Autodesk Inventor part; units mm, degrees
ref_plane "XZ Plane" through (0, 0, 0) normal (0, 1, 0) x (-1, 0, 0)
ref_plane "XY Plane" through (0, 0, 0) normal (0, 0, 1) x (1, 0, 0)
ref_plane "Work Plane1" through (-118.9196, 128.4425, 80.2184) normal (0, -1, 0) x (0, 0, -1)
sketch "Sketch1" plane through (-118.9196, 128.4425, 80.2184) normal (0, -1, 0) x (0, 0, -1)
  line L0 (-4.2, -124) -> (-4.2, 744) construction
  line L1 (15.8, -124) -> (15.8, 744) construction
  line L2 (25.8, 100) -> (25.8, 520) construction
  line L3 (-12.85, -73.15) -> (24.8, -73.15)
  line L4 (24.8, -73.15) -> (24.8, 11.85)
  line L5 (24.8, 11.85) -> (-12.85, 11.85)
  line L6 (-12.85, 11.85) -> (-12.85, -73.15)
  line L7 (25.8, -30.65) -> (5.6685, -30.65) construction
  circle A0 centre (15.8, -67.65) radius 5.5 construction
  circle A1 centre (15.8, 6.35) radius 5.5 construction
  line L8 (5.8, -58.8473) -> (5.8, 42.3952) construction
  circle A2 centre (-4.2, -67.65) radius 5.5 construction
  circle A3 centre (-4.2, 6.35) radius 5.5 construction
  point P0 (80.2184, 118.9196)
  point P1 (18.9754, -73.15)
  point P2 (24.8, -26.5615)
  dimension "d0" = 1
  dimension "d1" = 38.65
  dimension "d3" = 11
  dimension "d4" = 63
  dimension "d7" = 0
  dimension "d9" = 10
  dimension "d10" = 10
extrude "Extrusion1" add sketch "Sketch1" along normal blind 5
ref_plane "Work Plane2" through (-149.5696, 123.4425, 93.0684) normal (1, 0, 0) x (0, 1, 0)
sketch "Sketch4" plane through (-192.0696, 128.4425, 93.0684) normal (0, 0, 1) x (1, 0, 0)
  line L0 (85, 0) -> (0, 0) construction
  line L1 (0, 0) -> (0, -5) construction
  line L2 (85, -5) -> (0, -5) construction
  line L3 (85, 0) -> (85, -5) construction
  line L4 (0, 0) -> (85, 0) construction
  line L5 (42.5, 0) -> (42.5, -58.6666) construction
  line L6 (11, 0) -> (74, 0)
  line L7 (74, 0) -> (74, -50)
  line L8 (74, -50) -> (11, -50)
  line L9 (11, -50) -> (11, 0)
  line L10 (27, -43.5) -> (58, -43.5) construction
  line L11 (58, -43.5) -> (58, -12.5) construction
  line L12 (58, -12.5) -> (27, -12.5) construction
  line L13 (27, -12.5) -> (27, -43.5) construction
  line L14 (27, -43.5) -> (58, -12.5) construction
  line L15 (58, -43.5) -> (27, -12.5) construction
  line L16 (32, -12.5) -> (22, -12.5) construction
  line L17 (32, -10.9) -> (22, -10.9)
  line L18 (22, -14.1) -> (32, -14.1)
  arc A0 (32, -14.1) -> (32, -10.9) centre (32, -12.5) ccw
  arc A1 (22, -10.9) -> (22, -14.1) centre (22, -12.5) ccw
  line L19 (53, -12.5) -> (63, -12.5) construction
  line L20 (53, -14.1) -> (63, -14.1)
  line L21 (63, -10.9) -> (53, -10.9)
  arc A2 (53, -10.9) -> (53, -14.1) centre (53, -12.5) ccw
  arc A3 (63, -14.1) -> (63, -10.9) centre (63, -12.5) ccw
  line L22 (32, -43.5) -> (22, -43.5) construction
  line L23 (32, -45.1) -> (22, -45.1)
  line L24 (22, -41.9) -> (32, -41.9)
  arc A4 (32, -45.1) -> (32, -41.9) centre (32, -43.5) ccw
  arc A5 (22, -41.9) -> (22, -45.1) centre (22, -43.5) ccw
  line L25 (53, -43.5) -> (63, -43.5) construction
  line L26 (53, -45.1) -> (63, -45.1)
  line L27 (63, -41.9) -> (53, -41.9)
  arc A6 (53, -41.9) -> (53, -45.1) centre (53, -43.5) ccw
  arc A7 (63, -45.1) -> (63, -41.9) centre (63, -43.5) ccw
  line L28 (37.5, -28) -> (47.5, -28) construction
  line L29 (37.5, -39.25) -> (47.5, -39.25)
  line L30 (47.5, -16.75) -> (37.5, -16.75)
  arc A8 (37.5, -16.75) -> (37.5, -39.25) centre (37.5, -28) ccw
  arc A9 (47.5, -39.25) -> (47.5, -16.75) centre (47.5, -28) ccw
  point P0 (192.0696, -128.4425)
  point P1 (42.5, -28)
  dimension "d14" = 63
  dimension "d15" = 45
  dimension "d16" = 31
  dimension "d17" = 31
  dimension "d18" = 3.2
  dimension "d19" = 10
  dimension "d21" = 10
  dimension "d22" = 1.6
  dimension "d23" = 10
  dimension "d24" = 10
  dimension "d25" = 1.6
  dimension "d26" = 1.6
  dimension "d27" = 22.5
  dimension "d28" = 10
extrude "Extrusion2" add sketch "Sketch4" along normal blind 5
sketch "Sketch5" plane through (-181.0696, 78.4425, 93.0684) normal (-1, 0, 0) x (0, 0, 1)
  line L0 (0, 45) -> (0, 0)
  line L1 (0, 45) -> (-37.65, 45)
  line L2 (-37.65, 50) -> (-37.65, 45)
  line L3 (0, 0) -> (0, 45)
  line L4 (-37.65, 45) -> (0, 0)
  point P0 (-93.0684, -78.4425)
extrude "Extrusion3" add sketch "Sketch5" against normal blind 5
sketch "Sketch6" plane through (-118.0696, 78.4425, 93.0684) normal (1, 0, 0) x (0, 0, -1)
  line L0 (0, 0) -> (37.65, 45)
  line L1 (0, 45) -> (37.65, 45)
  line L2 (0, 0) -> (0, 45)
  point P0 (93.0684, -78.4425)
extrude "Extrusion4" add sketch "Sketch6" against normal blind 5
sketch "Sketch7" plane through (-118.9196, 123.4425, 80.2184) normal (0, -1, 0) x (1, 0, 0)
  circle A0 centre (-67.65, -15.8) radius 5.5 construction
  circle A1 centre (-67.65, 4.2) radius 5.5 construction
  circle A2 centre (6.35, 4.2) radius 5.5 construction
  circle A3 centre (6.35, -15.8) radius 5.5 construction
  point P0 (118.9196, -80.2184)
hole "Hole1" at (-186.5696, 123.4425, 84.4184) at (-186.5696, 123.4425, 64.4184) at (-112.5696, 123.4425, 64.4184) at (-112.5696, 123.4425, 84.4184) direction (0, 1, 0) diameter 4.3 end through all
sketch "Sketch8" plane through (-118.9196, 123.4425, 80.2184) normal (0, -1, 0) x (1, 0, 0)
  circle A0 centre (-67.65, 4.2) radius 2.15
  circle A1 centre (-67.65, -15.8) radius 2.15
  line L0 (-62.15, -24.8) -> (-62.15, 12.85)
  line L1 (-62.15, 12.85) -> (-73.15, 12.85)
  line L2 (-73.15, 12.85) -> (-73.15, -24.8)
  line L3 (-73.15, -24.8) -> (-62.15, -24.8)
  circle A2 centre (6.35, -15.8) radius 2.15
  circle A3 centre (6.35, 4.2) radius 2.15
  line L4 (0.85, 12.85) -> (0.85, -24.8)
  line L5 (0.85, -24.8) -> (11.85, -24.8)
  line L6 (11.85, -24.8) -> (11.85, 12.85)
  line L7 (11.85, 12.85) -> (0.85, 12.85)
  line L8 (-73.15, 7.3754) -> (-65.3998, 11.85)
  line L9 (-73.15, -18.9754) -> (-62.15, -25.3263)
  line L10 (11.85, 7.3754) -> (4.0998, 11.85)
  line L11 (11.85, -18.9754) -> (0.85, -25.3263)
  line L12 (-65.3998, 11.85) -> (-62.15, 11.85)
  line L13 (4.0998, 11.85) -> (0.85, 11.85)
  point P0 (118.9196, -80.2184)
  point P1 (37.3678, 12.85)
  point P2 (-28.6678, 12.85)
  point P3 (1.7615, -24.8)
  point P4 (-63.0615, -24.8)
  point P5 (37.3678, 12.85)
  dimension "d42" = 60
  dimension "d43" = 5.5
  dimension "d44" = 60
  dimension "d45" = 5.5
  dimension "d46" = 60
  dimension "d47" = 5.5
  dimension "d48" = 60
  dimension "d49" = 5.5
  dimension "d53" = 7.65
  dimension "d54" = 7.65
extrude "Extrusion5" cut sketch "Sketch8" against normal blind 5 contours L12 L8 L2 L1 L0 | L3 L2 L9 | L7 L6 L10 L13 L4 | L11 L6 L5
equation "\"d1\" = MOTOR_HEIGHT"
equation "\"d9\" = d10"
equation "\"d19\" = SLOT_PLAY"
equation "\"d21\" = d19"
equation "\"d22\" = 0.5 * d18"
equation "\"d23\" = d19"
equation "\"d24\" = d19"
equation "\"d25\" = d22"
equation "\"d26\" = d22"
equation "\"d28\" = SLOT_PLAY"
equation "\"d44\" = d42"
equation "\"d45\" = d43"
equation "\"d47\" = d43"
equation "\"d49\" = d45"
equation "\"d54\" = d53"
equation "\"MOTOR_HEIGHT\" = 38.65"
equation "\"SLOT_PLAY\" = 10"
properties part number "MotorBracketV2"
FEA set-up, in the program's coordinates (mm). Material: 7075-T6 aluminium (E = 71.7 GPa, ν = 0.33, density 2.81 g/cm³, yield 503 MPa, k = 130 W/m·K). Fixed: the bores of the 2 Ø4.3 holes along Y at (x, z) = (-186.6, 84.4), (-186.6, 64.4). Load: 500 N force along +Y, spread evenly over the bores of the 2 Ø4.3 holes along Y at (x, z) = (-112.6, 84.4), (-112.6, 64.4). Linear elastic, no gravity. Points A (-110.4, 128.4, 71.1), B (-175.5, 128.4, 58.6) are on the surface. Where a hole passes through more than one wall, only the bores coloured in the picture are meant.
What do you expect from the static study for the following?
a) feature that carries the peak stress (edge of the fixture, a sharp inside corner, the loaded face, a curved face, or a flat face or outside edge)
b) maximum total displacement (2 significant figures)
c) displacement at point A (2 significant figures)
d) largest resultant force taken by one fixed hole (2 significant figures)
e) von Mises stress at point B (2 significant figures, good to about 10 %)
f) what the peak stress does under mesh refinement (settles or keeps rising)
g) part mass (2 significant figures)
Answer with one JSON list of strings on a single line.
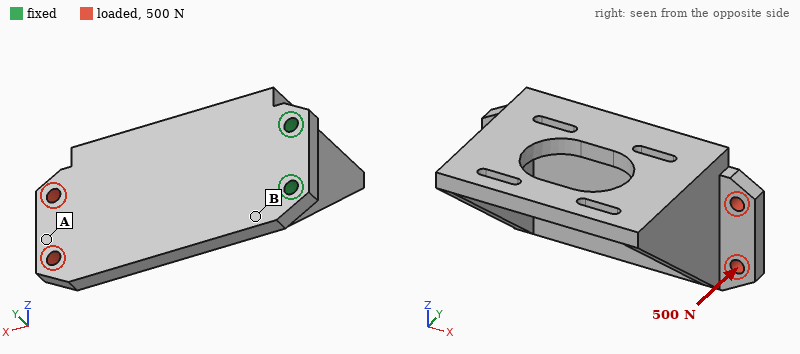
["edge of the fixture", "1.2 mm", "1.2 mm", "280 N", "91 MPa", "keeps rising", "100 g"]
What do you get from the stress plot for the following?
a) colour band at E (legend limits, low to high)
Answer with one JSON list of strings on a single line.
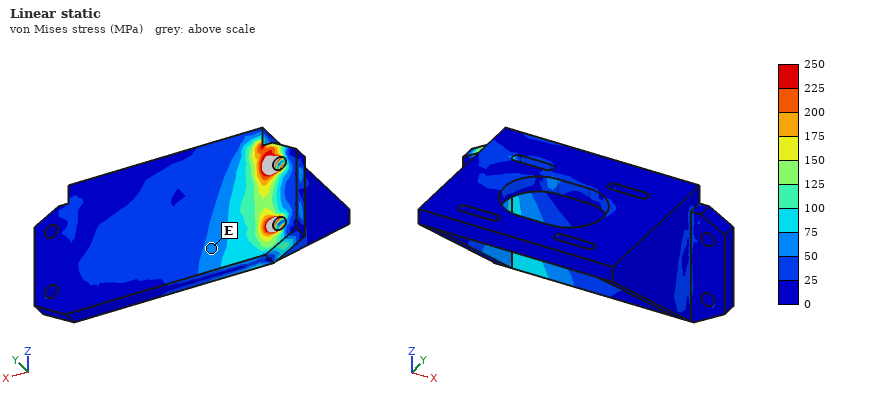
["50 to 75 MPa"]
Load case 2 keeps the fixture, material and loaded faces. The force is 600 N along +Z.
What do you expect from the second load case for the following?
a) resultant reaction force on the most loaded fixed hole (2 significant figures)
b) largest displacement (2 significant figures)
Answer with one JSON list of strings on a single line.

["2.0 kN", "72 µm"]
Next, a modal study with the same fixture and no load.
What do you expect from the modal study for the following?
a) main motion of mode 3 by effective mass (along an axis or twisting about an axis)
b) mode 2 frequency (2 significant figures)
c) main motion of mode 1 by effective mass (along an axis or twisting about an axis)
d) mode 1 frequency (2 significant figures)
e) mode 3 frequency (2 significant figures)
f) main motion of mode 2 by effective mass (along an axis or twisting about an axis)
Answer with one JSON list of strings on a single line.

["along Z", "1500 Hz", "along Y", "550 Hz", "3000 Hz", "along Z"]
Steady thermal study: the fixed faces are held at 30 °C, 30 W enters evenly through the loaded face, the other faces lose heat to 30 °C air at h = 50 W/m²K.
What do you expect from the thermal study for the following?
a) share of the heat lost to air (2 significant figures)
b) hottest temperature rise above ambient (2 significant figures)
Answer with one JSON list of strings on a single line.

["51 %", "50 K"]
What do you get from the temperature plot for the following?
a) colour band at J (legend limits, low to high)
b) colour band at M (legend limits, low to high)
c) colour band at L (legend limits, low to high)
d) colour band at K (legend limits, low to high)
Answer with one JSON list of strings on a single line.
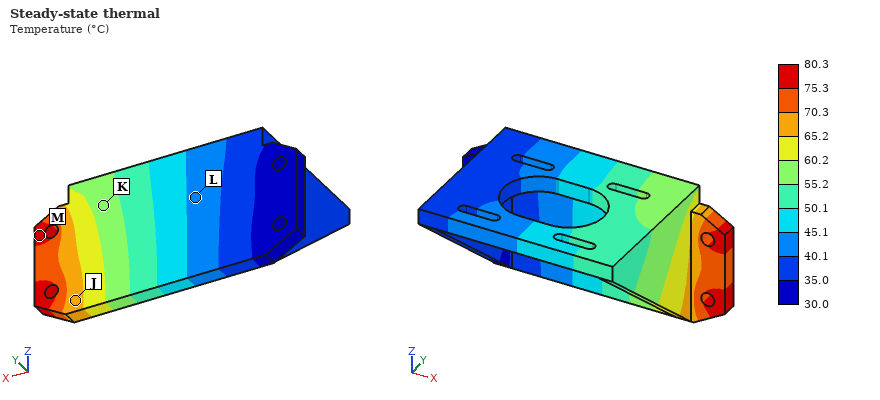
["65.2 to 70.3 °C", "75.3 to 80.3 °C", "40.1 to 45.1 °C", "55.2 to 60.2 °C"]
